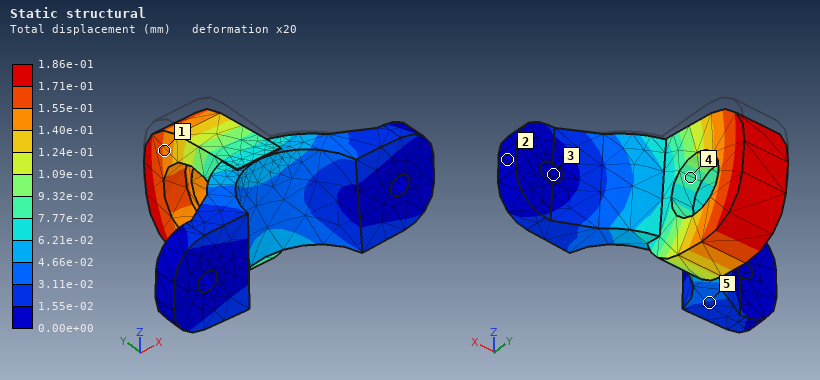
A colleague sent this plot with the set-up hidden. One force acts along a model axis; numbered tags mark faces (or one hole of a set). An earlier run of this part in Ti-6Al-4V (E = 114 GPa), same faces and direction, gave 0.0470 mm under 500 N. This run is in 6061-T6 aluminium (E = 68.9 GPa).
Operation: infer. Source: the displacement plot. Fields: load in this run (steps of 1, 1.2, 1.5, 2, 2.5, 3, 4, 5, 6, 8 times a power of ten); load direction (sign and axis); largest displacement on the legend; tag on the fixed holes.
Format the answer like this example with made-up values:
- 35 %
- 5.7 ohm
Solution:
- 1.2 kN
- -Z
- 1.86e-01 mm
- 3
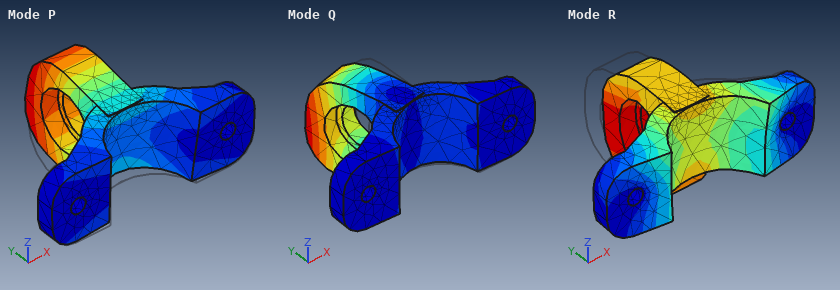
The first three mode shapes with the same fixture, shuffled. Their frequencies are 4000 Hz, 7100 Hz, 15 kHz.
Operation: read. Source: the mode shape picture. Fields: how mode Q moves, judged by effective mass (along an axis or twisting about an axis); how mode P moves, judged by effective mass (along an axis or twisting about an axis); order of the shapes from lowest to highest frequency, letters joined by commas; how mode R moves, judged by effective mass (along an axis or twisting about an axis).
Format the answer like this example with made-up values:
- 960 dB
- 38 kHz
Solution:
- along X
- along Z
- P, Q, R
- along Y
